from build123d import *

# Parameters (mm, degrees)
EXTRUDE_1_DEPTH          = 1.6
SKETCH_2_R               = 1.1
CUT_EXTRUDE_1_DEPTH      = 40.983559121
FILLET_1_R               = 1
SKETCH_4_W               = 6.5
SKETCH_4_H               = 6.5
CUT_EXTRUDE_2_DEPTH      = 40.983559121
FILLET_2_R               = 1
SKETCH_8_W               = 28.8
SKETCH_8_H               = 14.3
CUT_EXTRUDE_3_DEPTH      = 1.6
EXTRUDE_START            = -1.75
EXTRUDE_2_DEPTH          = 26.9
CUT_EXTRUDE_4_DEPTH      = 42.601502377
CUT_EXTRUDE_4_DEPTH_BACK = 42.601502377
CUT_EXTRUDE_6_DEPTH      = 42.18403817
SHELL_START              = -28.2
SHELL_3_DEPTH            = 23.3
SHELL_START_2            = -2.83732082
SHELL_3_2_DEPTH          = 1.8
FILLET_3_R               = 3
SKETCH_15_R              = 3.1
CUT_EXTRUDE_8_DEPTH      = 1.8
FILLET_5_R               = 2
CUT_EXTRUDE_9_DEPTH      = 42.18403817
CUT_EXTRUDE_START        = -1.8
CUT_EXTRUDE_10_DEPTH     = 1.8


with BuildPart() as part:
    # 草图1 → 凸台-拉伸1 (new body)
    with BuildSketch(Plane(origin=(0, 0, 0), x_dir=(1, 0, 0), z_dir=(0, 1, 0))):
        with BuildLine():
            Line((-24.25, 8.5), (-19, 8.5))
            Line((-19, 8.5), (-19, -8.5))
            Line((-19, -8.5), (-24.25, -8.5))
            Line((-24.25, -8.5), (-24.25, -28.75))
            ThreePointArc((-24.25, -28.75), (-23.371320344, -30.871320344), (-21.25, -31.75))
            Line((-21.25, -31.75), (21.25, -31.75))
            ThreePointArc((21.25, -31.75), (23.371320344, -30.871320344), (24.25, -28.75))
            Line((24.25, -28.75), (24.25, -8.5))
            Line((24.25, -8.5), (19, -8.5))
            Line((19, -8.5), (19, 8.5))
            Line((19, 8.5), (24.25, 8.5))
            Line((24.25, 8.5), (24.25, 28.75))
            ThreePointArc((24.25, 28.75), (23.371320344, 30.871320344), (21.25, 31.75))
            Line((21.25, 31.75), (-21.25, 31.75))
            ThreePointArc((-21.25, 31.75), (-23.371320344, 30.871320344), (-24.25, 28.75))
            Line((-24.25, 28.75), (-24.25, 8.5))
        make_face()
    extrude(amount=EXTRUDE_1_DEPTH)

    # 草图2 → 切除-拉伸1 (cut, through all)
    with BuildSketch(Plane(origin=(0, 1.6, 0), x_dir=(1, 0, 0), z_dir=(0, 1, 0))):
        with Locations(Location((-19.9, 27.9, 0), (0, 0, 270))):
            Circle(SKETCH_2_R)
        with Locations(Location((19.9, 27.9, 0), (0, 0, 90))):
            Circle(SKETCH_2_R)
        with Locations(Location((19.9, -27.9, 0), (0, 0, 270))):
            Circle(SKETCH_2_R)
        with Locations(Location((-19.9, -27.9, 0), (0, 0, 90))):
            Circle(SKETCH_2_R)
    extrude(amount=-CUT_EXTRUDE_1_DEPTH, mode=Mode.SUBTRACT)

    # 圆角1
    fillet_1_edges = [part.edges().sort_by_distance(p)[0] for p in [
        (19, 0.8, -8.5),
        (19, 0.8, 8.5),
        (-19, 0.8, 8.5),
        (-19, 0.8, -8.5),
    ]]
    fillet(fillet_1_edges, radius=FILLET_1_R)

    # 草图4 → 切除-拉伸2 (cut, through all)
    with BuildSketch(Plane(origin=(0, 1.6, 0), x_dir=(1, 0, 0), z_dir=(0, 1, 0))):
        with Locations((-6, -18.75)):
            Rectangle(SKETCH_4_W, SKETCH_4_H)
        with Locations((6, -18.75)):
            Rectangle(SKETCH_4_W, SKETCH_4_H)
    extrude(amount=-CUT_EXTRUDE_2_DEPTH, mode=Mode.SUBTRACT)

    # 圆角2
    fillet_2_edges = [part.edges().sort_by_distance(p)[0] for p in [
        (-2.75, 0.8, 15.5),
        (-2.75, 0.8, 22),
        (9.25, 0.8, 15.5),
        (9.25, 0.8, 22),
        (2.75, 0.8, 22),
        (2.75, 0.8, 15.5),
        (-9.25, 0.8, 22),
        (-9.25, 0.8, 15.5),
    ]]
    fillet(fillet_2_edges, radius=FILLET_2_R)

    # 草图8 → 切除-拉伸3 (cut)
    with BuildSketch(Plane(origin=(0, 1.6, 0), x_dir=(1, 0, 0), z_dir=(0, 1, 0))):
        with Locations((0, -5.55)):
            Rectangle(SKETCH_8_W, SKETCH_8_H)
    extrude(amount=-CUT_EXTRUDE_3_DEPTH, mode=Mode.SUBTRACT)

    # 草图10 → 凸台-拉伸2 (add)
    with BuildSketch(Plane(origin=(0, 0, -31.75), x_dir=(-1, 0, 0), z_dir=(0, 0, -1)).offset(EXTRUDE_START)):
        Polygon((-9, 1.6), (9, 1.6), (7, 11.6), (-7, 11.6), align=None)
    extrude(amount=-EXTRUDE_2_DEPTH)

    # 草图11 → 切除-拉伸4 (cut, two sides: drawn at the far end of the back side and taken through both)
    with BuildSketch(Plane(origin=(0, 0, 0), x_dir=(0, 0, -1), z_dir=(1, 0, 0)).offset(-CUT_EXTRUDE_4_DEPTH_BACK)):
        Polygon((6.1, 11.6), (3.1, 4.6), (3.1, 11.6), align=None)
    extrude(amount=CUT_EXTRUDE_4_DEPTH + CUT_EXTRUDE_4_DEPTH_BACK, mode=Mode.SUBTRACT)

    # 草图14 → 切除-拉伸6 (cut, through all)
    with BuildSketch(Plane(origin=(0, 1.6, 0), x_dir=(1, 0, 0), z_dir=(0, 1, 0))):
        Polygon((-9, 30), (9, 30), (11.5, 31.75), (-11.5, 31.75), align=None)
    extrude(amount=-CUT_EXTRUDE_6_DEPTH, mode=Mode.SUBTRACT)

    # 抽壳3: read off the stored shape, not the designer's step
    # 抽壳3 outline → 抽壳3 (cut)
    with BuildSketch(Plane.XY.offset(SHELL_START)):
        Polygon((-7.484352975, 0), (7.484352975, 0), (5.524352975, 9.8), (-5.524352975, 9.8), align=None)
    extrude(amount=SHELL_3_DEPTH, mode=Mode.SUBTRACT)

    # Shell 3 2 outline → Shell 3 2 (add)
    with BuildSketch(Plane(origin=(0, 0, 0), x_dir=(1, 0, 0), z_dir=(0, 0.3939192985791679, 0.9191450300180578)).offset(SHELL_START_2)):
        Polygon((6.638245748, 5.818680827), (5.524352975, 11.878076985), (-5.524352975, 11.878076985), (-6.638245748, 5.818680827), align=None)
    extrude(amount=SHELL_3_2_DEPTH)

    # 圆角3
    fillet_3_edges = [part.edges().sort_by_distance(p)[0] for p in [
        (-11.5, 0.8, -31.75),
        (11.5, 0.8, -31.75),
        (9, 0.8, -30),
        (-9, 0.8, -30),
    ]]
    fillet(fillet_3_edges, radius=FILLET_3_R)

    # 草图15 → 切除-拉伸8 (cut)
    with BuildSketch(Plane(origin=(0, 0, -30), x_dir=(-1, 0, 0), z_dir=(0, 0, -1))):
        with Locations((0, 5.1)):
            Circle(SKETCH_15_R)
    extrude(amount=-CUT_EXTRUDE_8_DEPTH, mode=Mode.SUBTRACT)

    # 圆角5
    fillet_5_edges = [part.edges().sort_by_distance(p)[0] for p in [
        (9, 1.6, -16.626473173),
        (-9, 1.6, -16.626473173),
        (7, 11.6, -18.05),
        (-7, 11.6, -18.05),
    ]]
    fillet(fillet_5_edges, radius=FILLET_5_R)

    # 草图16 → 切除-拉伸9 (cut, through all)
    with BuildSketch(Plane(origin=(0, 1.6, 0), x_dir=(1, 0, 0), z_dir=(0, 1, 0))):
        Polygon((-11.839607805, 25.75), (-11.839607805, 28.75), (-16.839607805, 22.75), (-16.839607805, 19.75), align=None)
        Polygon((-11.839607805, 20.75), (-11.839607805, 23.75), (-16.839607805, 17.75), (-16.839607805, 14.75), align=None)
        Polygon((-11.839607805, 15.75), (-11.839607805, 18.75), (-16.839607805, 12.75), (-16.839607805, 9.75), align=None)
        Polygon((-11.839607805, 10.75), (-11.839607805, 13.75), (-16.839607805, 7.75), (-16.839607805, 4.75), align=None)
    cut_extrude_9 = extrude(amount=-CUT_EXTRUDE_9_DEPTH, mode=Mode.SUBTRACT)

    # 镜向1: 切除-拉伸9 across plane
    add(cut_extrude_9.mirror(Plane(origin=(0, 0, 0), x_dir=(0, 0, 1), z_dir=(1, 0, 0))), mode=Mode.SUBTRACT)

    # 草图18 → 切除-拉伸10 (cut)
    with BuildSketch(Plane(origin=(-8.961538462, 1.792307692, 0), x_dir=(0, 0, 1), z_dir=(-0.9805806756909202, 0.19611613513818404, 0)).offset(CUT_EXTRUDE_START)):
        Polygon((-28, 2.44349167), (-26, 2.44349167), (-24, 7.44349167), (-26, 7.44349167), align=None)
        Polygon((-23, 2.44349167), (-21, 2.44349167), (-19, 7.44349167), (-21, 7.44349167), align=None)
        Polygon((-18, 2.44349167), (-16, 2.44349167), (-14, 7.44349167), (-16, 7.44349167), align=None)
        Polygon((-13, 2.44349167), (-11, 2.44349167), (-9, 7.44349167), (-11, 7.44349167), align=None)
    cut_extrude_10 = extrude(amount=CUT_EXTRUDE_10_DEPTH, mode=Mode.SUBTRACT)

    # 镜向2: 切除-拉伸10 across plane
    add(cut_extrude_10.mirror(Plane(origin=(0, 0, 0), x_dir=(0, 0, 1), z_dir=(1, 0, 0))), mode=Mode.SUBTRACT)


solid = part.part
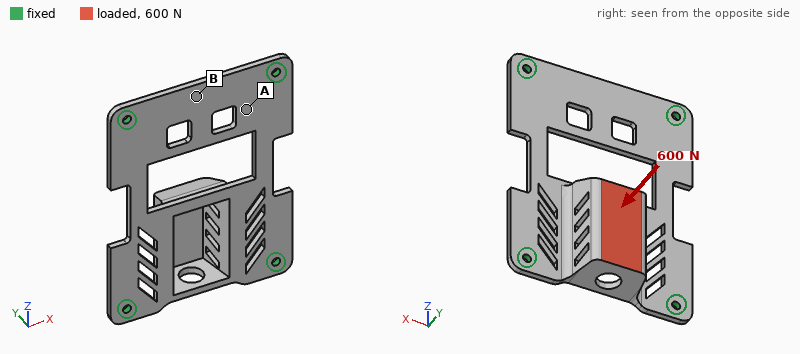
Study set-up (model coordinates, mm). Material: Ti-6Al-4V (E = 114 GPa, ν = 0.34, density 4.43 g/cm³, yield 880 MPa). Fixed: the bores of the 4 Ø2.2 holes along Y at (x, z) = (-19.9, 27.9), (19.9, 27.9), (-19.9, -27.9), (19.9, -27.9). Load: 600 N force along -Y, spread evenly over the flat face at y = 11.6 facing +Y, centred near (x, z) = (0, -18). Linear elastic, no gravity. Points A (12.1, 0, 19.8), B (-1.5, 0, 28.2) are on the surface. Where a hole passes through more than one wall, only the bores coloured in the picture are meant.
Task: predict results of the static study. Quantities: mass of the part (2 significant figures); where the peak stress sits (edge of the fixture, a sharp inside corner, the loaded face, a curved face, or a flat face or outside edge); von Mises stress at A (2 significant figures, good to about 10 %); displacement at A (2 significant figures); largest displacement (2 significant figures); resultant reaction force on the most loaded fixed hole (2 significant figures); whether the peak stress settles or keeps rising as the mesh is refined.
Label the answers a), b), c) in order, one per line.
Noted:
a) 20 g
b) edge of the fixture
c) 64 MPa
d) 0.068 mm
e) 0.41 mm
f) 290 N
g) keeps rising
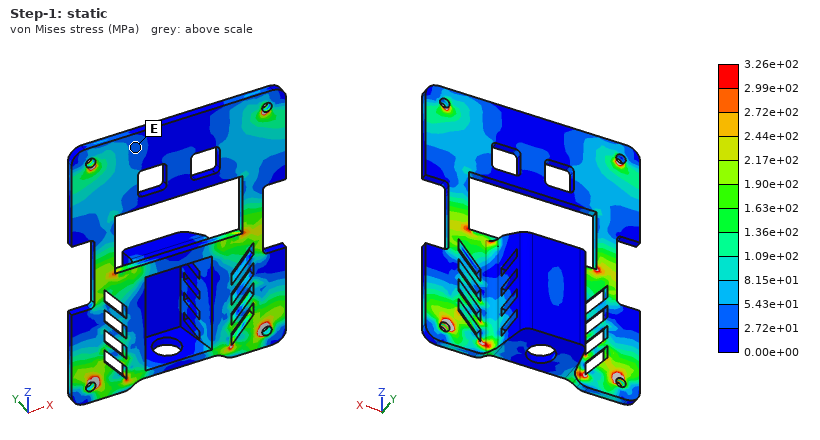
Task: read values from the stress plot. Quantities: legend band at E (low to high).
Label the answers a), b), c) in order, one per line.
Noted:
a) 2.72e+01 to 5.43e+01 MPa
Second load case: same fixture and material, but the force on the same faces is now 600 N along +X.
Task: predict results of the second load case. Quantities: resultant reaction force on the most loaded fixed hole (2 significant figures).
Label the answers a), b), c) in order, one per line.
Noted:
a) 360 N
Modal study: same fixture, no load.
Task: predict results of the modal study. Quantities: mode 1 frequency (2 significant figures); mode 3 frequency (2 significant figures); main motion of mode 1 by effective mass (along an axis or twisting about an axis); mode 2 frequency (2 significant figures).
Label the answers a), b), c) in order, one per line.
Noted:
a) 1700 Hz
b) 4500 Hz
c) along Y
d) 4200 Hz
